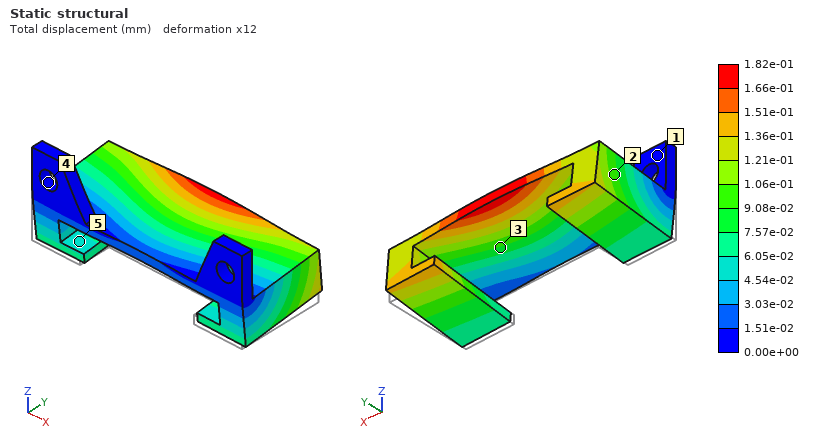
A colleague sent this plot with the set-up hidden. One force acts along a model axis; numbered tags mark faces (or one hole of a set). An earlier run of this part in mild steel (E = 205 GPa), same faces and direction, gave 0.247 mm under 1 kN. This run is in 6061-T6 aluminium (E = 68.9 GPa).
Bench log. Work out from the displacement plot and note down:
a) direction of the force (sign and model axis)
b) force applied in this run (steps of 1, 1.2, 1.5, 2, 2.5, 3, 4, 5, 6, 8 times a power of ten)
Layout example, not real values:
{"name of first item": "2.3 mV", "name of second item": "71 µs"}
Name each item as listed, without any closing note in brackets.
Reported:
{"direction of the force": "+Z", "force applied in this run": "250 N"}
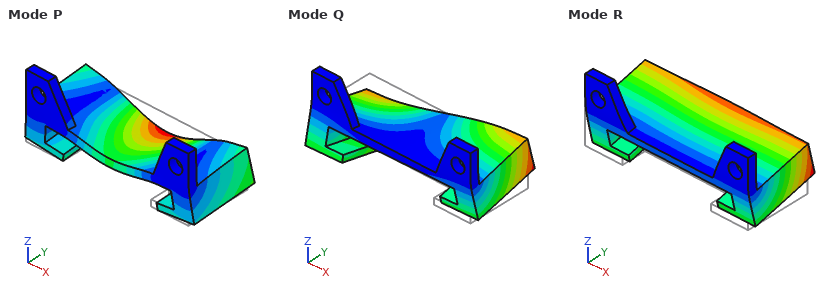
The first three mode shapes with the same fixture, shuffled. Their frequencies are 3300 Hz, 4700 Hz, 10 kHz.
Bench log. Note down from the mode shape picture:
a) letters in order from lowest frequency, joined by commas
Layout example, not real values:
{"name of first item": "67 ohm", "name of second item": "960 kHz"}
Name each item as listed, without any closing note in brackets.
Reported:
{"letters in order from lowest frequency, joined by commas": "R, Q, P"}
